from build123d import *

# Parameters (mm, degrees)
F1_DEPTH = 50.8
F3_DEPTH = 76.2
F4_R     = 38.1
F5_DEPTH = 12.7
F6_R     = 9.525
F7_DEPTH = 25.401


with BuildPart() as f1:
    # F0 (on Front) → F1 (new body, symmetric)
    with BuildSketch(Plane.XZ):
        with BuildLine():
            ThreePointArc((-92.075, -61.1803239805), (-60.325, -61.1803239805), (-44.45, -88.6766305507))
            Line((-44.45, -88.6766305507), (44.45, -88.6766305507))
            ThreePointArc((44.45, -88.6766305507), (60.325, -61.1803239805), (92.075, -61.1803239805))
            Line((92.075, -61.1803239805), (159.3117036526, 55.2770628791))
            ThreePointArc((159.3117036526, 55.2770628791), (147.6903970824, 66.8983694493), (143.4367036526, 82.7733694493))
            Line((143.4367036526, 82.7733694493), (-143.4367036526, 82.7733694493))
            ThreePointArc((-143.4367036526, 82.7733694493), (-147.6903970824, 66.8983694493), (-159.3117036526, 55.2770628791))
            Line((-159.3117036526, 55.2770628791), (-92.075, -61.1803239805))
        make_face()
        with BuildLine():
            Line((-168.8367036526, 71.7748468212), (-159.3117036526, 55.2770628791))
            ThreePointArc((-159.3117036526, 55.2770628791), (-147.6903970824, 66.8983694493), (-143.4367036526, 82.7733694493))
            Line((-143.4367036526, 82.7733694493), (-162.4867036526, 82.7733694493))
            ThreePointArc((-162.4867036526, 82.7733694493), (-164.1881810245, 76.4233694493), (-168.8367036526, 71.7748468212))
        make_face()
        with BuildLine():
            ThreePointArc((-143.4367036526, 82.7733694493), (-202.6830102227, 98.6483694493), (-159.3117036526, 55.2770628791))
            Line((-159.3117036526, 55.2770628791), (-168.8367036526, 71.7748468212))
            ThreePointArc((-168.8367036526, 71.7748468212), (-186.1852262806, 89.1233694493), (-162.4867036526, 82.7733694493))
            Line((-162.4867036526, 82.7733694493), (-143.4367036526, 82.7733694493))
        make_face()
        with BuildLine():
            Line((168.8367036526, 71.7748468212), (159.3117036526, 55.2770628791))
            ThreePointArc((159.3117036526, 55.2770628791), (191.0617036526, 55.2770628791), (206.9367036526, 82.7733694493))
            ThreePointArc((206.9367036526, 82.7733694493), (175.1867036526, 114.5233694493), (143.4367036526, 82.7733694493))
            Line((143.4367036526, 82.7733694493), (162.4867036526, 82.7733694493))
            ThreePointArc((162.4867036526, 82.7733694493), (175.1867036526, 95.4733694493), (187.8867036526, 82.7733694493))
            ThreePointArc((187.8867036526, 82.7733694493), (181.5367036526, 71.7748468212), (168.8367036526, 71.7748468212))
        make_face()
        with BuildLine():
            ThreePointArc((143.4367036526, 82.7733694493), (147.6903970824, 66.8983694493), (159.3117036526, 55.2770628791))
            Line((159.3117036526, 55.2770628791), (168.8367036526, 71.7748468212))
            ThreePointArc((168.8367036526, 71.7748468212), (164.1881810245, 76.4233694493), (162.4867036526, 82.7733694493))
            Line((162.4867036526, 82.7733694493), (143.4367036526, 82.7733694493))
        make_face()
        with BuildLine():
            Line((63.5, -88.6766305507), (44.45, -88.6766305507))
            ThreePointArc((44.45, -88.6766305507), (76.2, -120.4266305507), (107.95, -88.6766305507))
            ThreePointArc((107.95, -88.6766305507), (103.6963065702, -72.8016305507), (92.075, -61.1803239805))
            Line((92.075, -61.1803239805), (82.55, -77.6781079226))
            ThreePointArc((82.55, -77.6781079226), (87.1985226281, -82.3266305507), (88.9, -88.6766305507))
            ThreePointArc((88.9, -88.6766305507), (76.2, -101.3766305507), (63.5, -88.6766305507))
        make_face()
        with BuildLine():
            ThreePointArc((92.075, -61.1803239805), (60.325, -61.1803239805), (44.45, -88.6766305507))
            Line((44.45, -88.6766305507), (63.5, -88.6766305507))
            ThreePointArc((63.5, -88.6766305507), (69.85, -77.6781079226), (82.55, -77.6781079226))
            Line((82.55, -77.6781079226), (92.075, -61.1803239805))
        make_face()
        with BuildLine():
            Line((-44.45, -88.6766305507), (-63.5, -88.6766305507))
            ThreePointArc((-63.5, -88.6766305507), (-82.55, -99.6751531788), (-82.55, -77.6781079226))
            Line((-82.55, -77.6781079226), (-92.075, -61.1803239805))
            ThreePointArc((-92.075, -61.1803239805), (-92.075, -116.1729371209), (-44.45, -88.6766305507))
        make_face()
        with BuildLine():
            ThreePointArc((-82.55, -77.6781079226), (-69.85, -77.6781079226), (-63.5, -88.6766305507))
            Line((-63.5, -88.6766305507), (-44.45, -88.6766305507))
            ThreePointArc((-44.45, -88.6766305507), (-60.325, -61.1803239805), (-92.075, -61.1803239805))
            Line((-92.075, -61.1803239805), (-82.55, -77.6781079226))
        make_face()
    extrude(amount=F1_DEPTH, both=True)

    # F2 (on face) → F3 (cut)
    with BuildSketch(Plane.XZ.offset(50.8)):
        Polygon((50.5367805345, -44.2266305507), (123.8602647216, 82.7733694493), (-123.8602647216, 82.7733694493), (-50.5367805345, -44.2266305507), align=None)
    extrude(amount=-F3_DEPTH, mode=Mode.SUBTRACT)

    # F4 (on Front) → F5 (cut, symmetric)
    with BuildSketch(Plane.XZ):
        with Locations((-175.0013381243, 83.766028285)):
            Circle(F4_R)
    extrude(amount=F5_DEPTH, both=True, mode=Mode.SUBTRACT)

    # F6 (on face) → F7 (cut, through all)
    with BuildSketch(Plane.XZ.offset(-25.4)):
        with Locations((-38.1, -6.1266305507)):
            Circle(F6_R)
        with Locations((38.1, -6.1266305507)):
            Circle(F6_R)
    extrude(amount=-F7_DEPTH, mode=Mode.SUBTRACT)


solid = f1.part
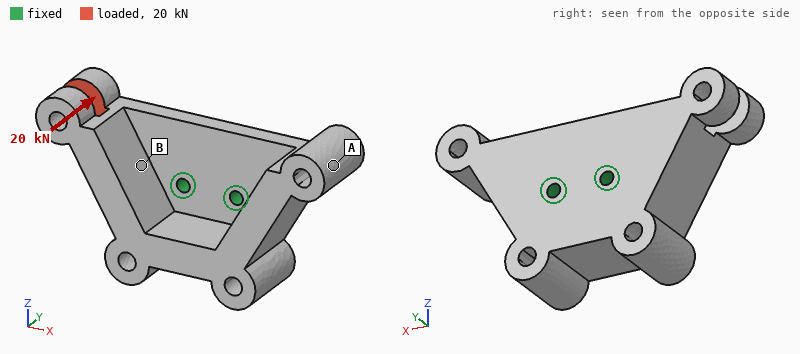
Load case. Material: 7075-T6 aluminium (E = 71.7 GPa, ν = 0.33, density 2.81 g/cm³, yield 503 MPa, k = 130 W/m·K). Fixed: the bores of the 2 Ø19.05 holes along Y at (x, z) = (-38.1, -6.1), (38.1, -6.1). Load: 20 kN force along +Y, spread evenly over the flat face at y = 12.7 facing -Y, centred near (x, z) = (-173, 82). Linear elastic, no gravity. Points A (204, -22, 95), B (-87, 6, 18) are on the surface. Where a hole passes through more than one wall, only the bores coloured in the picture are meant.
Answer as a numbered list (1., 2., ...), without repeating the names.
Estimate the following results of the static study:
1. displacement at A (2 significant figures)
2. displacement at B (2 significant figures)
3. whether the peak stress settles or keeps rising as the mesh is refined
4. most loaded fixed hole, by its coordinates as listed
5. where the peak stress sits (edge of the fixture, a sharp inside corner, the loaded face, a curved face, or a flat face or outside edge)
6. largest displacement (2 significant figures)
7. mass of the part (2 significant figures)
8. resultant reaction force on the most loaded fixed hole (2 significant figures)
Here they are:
1. 0.15 mm
2. 0.19 mm
3. keeps rising
4. (-38.1, -6.1)
5. edge of the fixture
6. 0.84 mm
7. 9.5 kg
8. 42 kN
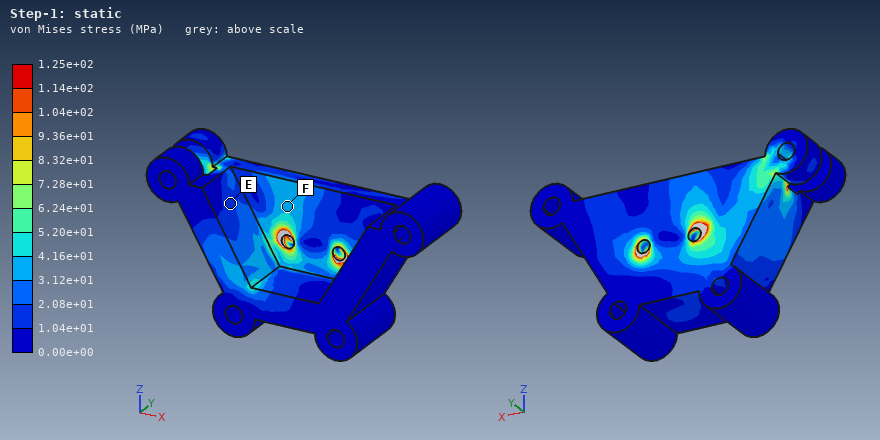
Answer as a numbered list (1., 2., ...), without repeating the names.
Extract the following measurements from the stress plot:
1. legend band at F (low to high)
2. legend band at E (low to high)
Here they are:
1. 3.12e+01 to 4.16e+01 MPa
2. 1.04e+01 to 2.08e+01 MPa
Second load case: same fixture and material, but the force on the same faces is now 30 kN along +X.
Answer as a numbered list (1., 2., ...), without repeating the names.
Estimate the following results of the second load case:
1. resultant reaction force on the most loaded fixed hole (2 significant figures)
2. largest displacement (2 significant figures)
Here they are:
1. 33 kN
2. 0.51 mm
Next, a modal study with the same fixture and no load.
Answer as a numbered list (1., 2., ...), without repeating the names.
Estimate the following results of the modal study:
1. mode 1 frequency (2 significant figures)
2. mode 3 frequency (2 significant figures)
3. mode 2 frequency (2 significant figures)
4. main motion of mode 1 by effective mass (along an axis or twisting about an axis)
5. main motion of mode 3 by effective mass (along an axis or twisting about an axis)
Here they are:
1. 650 Hz
2. 1100 Hz
3. 800 Hz
4. along Z
5. twisting about Y
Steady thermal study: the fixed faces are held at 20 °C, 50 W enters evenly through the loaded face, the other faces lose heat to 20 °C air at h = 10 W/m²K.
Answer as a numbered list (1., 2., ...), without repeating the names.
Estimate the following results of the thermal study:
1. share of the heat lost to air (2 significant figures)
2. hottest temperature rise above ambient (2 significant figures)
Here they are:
1. 18 %
2. 23 K
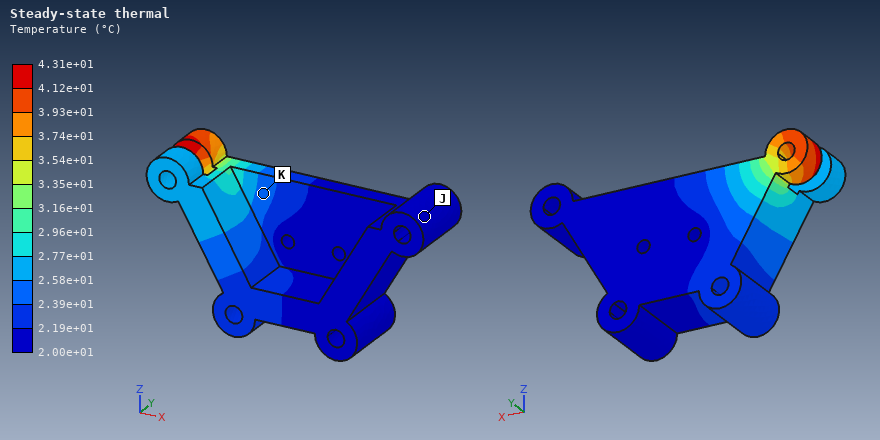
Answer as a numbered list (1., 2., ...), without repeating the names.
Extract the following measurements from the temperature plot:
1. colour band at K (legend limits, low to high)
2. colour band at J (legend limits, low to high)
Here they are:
1. 2.39e+01 to 2.58e+01 °C
2. 2.00e+01 to 2.19e+01 °C
